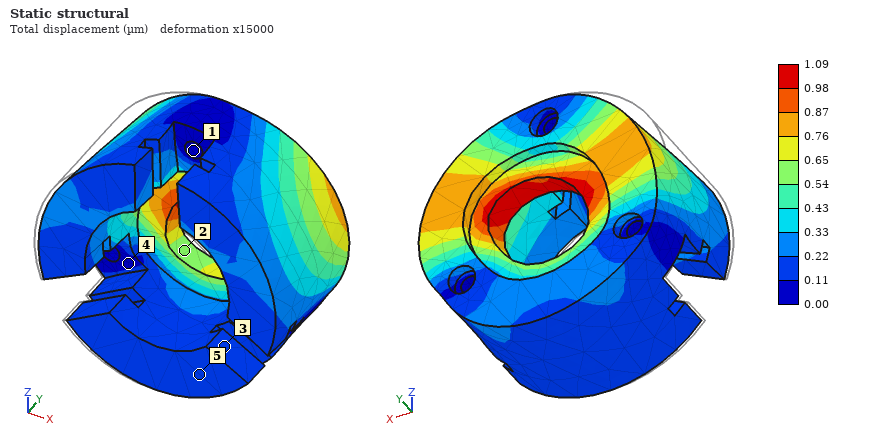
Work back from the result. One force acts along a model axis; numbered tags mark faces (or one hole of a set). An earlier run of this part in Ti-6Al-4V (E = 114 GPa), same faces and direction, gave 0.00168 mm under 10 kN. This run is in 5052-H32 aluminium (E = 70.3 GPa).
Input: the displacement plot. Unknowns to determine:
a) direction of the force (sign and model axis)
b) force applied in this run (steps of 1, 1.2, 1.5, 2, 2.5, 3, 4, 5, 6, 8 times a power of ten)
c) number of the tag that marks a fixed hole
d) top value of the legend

+X
4 kN
1
1.09 µm
